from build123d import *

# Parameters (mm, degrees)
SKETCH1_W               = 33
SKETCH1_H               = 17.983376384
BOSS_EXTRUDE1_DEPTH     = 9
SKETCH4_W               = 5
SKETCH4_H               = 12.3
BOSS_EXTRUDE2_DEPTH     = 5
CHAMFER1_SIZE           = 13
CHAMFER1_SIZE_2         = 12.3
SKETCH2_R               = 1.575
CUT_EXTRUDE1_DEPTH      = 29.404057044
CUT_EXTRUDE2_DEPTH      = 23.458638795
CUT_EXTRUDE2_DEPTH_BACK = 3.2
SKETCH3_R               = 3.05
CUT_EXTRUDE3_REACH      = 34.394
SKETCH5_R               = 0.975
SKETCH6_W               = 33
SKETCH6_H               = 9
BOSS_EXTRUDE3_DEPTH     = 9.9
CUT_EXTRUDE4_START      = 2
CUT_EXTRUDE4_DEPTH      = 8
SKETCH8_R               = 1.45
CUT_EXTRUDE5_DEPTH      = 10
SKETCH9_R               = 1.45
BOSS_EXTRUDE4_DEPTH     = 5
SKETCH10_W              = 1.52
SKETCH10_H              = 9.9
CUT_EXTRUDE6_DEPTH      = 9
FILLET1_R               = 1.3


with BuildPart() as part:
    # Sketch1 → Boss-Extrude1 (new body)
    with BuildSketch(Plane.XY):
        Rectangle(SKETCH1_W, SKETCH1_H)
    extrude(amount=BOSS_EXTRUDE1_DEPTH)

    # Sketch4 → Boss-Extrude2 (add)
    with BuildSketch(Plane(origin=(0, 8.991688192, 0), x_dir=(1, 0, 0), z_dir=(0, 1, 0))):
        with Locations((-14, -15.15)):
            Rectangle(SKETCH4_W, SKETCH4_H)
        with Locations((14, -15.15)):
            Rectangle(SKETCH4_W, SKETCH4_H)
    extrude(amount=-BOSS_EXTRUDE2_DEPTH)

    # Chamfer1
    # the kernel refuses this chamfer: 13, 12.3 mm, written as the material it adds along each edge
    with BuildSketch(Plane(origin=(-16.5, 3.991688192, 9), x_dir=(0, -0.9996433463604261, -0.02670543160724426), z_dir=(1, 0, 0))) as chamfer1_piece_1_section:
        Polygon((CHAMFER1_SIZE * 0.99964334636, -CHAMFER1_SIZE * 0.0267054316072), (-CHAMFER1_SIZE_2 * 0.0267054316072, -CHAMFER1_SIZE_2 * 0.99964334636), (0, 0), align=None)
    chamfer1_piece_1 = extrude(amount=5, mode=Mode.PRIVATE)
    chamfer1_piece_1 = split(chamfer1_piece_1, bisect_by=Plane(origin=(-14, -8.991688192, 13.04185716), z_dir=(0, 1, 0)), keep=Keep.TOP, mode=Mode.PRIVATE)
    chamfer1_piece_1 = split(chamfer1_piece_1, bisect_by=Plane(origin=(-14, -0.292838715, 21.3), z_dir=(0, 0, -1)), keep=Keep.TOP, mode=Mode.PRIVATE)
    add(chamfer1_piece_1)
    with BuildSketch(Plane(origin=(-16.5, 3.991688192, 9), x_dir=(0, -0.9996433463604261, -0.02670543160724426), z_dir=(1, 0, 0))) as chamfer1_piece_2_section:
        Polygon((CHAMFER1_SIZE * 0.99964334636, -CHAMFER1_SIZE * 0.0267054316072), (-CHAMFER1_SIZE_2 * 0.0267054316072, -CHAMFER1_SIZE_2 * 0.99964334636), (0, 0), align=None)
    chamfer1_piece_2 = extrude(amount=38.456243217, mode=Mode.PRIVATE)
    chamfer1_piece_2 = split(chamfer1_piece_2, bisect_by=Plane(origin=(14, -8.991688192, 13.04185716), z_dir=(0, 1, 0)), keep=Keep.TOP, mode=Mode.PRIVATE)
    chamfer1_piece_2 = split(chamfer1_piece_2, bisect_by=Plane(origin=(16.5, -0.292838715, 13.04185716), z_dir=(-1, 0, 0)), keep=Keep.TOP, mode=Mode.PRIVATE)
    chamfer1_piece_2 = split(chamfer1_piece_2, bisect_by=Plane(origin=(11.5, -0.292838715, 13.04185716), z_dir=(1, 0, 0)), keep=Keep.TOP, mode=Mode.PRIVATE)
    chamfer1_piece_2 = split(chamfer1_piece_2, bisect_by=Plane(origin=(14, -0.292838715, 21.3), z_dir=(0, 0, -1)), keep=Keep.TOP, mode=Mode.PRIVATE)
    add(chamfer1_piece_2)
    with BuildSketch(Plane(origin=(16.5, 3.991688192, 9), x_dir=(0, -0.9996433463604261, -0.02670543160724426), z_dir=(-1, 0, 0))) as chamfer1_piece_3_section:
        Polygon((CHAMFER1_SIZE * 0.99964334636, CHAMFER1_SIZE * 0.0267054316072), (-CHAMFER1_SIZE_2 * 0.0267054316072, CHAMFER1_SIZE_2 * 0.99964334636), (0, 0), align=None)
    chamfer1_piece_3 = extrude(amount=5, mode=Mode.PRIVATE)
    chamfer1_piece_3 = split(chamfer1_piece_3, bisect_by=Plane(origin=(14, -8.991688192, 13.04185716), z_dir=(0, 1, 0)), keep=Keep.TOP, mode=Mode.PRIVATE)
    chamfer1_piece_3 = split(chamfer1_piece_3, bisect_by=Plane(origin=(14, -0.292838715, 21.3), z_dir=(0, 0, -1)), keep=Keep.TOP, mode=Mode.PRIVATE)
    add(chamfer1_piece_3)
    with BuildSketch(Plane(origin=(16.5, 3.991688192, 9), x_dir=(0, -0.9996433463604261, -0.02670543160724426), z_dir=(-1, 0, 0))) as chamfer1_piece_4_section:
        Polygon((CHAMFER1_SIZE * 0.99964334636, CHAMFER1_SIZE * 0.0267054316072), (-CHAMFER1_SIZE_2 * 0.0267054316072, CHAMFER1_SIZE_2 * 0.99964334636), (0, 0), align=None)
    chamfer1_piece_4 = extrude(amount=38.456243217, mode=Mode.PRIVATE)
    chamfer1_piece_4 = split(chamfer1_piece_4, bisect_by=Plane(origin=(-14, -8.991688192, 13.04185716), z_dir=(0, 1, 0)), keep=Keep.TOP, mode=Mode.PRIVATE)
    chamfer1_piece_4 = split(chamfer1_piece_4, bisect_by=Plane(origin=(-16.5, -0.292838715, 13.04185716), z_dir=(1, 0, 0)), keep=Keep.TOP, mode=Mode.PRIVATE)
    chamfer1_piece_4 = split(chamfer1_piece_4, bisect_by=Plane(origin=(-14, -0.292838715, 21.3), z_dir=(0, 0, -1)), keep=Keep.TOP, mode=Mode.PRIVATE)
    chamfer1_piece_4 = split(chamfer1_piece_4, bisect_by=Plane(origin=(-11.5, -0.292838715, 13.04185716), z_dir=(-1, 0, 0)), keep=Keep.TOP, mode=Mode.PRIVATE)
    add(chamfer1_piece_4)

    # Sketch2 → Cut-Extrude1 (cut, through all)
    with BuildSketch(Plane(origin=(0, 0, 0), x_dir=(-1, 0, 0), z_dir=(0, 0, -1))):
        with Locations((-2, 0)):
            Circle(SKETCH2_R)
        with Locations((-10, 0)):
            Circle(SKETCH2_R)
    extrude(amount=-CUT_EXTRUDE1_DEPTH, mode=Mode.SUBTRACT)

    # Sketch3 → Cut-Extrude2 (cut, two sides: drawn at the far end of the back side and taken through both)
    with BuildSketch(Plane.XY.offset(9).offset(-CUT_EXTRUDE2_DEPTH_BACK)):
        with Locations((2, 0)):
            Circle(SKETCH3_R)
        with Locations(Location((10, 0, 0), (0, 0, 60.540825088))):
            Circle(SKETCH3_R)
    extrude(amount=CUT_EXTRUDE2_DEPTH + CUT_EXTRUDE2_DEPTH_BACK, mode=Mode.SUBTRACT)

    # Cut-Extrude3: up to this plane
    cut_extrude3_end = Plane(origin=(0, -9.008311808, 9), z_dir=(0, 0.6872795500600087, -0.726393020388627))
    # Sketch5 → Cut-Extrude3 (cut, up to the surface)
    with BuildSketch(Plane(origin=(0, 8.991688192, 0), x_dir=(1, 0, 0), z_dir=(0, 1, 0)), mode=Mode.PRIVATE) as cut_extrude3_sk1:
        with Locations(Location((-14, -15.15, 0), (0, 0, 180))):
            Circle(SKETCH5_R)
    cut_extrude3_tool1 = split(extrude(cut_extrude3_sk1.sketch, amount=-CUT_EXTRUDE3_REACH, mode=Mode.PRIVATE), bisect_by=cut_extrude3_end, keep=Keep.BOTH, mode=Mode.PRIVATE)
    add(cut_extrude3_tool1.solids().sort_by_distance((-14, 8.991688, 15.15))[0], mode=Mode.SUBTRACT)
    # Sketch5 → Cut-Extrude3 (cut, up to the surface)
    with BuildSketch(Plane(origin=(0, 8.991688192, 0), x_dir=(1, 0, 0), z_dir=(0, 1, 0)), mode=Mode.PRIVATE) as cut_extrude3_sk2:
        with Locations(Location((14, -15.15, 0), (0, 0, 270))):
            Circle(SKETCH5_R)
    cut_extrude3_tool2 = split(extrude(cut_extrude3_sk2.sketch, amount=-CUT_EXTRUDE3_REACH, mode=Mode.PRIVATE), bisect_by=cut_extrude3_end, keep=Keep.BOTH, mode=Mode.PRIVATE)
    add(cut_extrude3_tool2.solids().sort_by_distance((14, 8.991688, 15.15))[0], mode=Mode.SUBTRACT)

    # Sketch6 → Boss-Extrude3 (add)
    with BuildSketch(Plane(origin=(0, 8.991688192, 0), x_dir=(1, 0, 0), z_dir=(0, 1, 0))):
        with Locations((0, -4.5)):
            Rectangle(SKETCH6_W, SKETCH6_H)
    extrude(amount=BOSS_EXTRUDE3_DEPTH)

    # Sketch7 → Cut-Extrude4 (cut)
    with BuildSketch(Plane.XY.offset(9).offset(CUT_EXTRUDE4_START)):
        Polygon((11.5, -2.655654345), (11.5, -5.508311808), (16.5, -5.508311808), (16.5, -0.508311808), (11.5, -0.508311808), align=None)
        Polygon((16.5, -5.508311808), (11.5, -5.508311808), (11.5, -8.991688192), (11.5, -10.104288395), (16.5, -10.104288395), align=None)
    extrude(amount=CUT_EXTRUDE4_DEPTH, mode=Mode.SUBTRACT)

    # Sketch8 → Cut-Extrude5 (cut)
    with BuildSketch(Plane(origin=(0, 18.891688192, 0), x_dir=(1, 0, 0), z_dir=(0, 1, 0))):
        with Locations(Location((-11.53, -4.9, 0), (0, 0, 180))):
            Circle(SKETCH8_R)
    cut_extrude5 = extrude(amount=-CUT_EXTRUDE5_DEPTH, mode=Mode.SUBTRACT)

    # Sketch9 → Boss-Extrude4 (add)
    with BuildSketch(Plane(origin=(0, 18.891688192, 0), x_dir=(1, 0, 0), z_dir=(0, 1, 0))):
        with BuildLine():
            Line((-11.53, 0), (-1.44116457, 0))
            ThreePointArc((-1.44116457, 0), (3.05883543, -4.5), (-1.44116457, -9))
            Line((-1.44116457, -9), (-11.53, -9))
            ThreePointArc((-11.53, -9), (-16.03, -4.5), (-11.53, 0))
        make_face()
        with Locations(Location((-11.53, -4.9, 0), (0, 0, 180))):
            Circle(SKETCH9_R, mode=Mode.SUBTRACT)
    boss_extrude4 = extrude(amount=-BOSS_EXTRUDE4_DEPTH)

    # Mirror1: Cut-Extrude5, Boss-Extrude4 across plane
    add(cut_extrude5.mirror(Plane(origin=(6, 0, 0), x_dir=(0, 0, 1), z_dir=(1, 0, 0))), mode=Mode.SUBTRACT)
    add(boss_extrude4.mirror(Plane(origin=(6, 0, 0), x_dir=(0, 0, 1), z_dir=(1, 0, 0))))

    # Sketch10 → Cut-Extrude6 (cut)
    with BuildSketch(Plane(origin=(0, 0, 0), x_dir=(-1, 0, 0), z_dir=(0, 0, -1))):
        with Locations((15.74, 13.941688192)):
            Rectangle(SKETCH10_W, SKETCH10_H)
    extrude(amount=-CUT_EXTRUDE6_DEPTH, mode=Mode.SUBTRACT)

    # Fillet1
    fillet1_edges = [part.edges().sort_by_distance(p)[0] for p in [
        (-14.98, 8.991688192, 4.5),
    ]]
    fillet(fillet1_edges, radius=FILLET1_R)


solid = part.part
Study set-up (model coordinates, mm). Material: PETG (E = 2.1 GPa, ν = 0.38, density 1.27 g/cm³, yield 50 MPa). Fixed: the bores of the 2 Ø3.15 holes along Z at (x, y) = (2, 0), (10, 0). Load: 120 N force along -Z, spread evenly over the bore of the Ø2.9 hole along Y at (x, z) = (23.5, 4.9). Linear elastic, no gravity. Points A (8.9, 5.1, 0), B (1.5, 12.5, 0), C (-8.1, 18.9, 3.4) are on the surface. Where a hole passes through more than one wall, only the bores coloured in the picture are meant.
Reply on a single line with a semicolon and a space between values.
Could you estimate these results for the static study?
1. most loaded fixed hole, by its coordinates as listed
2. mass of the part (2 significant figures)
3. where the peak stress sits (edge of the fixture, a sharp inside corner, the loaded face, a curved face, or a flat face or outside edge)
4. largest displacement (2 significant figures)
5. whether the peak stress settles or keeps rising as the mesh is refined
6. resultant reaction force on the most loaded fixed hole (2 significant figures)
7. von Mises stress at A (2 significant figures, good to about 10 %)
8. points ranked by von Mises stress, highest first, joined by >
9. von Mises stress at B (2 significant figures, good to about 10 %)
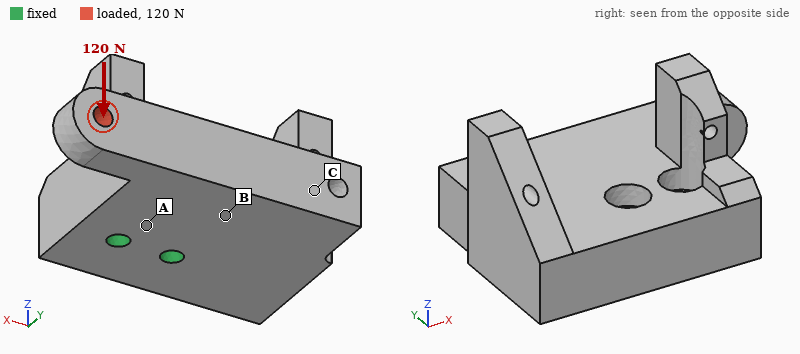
(10, 0); 12 g; edge of the fixture; 0.59 mm; keeps rising; 210 N; 8.4 MPa; A > B > C; 4.6 MPa
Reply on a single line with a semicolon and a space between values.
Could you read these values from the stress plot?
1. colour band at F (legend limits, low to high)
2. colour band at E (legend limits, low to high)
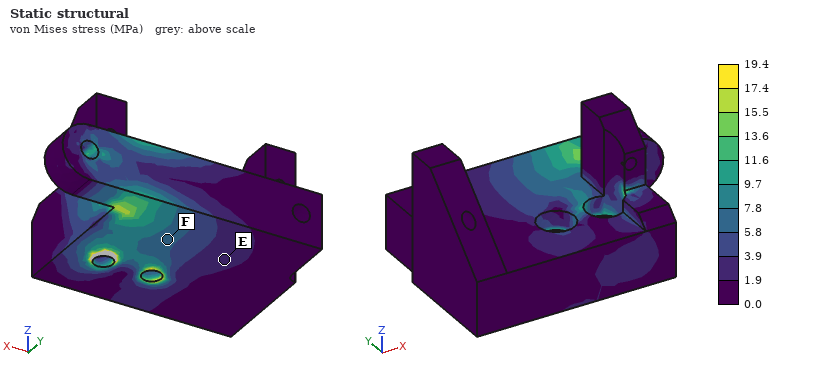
5.8 to 7.8 MPa; 1.9 to 3.9 MPa
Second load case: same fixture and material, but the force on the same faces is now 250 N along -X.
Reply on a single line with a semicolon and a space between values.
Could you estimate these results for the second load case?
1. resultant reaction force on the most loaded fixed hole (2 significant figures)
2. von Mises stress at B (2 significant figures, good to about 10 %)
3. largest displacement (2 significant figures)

410 N; 2.4 MPa; 0.22 mm
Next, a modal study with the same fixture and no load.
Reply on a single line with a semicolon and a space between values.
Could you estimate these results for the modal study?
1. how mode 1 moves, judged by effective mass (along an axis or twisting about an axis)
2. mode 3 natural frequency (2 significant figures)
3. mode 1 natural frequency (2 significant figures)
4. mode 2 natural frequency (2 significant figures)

along Z; 2800 Hz; 2200 Hz; 2400 Hz
